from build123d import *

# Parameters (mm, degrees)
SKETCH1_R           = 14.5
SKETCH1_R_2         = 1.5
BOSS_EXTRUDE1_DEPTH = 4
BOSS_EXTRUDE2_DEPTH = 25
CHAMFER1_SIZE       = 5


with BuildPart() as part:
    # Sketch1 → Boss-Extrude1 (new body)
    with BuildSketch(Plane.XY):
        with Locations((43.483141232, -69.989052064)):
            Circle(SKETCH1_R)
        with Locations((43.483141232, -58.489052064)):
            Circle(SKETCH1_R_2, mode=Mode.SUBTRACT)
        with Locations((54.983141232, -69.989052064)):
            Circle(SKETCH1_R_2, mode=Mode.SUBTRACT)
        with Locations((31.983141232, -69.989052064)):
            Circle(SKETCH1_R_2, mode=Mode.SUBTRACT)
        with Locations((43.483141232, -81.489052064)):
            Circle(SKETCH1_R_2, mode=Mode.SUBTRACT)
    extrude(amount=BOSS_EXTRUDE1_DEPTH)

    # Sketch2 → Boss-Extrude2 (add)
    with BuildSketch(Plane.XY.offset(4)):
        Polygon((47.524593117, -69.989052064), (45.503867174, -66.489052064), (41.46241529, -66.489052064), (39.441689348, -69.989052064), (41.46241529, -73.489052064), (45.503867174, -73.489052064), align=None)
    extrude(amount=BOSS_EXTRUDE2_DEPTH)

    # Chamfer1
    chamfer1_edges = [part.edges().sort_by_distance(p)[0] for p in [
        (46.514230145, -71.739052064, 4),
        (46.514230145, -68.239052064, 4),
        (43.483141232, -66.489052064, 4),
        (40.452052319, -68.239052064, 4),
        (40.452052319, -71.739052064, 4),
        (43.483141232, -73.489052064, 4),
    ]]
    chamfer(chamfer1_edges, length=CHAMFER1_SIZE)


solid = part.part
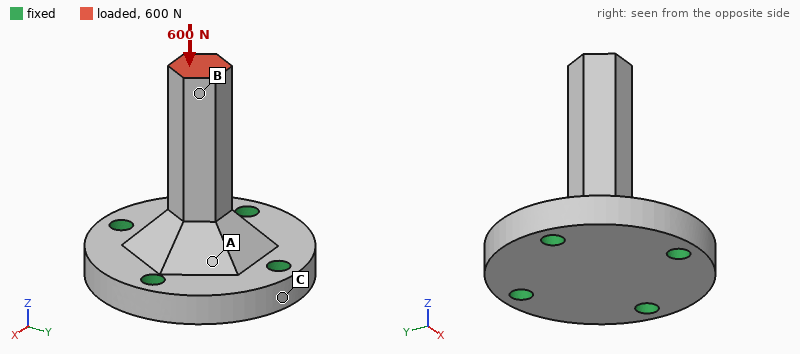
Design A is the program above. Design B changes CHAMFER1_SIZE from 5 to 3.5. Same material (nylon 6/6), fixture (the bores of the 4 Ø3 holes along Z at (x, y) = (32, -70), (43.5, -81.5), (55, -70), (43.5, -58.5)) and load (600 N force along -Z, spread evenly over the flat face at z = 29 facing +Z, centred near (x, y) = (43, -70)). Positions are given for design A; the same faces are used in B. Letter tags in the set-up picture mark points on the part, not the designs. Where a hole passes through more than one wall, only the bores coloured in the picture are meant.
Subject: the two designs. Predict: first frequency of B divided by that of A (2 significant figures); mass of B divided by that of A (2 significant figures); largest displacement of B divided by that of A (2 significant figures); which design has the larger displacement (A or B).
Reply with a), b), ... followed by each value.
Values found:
a) 0.88
b) 0.94
c) 1.1
d) B
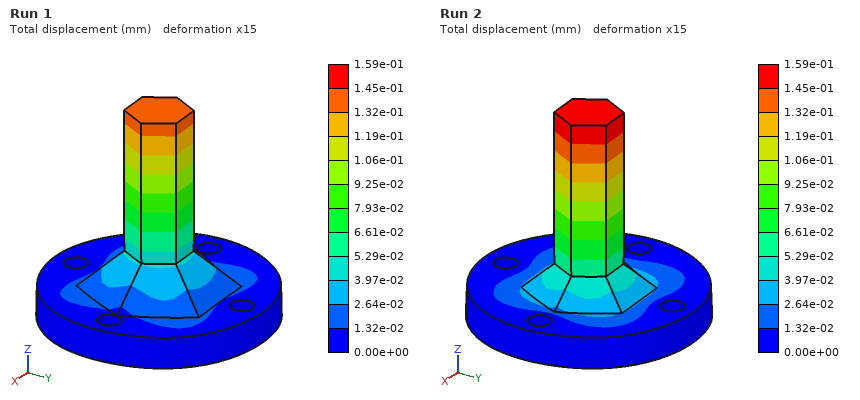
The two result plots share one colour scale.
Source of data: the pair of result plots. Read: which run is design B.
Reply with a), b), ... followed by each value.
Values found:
a) Run 2
